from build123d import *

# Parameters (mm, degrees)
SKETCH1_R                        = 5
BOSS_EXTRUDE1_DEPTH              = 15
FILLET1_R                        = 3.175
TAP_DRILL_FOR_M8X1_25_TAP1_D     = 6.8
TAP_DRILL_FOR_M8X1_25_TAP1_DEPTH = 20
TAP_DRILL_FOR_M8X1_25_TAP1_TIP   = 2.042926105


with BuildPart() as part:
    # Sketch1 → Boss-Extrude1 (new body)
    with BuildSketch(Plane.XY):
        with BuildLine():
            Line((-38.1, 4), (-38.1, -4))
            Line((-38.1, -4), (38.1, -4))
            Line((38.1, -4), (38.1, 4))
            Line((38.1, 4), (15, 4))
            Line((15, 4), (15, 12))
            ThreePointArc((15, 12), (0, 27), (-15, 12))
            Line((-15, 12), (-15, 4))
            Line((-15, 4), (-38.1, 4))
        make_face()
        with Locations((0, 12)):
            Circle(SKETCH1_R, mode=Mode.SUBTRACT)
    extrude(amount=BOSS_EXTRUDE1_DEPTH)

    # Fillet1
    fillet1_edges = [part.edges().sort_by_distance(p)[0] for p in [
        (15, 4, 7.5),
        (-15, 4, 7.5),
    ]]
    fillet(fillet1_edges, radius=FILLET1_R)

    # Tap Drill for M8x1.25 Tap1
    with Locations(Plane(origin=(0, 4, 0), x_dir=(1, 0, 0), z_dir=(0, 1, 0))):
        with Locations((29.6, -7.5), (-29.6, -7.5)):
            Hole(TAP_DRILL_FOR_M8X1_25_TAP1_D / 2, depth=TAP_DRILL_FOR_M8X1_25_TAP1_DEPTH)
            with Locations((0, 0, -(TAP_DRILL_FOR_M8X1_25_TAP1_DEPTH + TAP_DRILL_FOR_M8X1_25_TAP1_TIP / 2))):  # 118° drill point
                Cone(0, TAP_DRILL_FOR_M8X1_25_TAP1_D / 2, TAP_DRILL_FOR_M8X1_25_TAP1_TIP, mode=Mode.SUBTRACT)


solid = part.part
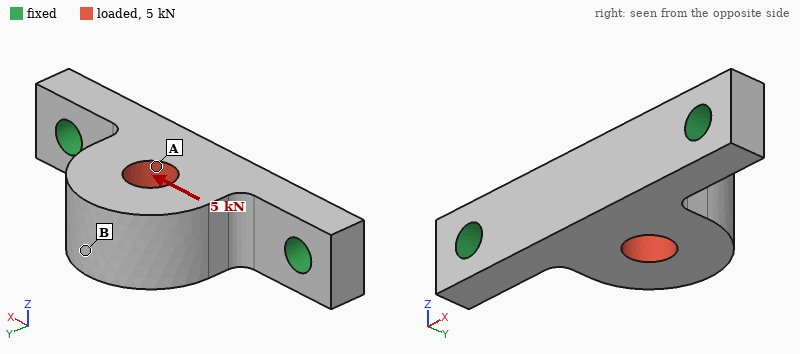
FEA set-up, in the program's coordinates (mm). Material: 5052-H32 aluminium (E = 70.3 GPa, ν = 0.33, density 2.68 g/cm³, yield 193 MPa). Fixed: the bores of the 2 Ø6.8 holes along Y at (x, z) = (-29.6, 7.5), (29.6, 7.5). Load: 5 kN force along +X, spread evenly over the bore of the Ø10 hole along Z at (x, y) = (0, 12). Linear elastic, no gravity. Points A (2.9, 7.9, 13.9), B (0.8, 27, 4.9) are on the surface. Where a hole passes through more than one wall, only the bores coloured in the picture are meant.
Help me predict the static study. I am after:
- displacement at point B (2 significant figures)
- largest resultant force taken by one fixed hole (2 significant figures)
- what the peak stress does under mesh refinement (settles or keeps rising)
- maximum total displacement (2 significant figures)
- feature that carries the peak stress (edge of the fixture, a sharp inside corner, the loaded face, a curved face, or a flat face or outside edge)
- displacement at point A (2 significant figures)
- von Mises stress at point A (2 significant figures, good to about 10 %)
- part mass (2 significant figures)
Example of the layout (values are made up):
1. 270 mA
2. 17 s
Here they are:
1. 27 µm
2. 2.8 kN
3. keeps rising
4. 27 µm
5. edge of the fixture
6. 11 µm
7. 30 MPa
8. 44 g
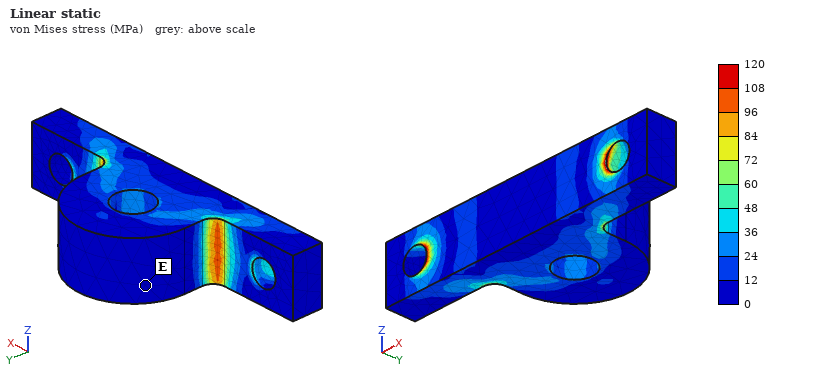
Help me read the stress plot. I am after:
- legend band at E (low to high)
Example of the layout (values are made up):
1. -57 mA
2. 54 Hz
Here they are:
1. 0 to 12 MPa
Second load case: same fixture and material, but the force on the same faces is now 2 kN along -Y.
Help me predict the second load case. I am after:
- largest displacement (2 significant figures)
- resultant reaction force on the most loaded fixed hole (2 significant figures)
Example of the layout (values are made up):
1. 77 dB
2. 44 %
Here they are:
1. 16 µm
2. 1.1 kN
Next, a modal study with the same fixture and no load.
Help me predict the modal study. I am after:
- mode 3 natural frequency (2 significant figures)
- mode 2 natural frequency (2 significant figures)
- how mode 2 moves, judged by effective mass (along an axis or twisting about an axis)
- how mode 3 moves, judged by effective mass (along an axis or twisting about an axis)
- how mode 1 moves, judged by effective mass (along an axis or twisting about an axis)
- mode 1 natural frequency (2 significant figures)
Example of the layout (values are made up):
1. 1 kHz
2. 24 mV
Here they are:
1. 14 kHz
2. 11 kHz
3. along Y
4. along X
5. along Z
6. 5000 Hz
